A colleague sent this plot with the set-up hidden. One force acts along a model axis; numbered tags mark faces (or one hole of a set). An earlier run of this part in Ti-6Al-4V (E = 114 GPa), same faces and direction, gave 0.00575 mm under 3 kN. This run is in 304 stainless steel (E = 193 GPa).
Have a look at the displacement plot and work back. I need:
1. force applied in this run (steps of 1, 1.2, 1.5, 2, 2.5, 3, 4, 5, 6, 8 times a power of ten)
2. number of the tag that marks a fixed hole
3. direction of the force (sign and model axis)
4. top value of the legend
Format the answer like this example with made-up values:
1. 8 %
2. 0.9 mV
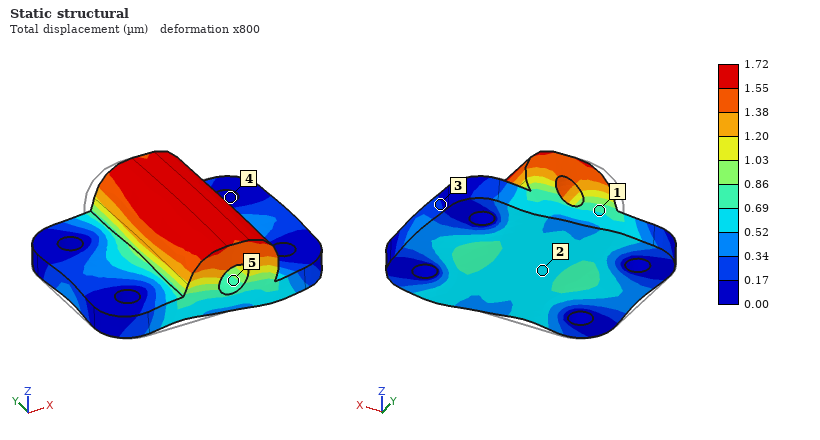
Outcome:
1. 1.5 kN
2. 4
3. +X
4. 1.72 µm
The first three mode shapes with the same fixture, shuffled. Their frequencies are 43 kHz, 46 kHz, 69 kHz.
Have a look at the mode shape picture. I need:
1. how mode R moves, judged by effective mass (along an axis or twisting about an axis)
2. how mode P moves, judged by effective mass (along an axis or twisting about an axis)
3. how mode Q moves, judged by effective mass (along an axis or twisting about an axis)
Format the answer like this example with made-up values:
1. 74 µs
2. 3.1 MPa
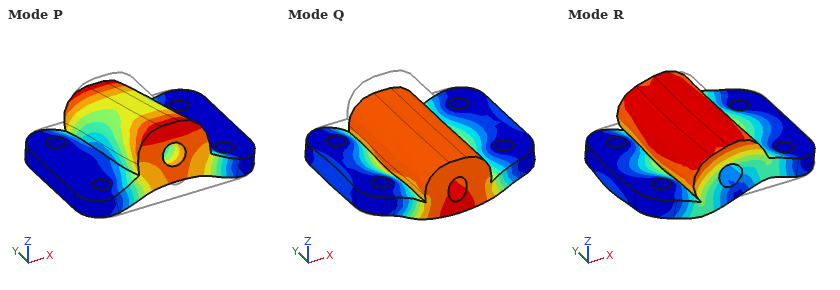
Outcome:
1. along X
2. along Y
3. along Z
